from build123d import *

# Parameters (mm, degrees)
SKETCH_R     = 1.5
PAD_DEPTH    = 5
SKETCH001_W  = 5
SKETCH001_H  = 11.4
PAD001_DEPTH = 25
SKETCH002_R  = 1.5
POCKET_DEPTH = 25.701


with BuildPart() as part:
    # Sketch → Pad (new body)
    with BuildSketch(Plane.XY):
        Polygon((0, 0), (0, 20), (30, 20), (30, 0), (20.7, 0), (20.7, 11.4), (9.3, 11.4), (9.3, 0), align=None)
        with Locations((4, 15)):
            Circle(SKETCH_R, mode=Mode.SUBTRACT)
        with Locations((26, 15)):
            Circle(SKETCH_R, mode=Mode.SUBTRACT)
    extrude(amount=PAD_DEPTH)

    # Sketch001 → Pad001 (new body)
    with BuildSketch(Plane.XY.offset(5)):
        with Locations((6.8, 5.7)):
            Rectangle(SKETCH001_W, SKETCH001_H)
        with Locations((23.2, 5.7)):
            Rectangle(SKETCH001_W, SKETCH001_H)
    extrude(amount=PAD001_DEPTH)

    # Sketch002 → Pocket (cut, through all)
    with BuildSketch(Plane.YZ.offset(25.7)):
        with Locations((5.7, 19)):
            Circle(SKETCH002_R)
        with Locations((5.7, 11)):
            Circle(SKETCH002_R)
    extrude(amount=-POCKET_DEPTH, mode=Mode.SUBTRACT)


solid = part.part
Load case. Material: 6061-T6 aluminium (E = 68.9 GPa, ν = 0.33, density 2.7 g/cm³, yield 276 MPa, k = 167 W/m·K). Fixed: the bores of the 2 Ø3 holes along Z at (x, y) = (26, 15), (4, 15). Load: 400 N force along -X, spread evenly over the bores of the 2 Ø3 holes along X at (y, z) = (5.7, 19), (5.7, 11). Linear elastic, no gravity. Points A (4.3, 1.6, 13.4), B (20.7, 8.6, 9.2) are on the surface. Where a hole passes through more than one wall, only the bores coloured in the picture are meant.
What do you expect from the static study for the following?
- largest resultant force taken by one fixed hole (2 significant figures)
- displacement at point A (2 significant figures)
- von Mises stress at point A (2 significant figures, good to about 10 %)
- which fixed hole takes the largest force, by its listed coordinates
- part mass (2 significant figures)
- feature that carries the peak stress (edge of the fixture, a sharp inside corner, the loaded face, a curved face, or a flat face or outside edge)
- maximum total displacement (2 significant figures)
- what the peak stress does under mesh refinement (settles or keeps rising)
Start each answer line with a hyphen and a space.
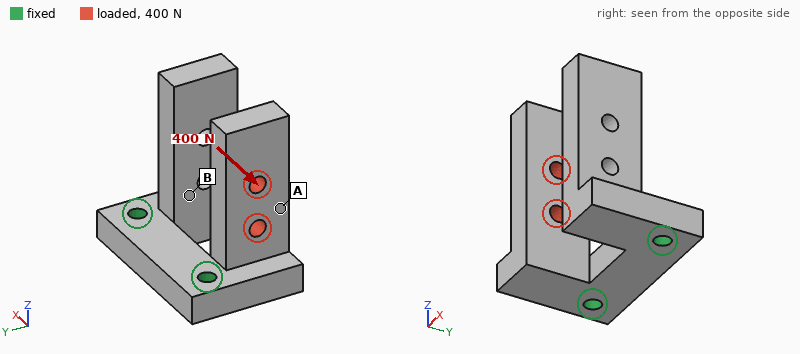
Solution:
- 380 N
- 0.074 mm
- 29 MPa
- (4, 15)
- 13 g
- a sharp inside corner
- 0.20 mm
- keeps rising
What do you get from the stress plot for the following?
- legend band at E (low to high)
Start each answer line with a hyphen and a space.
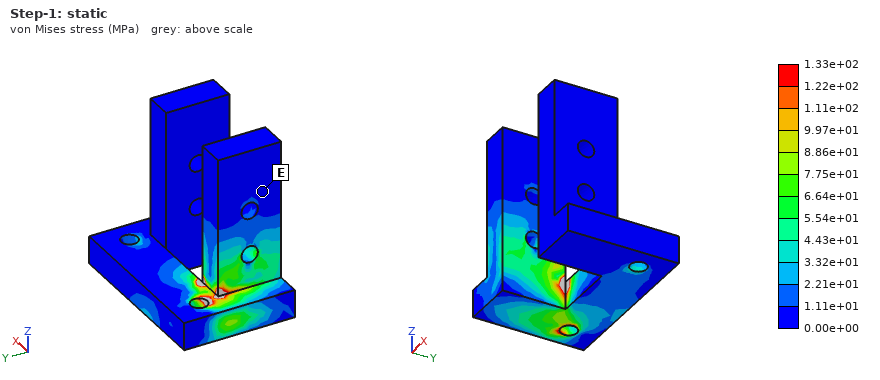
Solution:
- 0.00e+00 to 1.11e+01 MPa
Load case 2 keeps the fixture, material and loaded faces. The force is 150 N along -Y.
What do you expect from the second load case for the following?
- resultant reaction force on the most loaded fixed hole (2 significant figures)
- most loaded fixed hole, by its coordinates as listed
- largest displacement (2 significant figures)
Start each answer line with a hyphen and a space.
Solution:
- 140 N
- (4, 15)
- 59 µm
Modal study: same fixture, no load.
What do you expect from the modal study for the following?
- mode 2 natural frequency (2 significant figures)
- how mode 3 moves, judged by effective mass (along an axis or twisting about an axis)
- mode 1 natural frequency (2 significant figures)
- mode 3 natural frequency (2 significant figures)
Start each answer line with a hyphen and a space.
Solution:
- 3900 Hz
- along Y
- 3800 Hz
- 4400 Hz
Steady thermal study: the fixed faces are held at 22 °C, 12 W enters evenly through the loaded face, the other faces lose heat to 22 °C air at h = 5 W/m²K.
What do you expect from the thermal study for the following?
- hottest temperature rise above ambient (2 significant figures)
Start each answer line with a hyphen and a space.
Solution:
- 26 K
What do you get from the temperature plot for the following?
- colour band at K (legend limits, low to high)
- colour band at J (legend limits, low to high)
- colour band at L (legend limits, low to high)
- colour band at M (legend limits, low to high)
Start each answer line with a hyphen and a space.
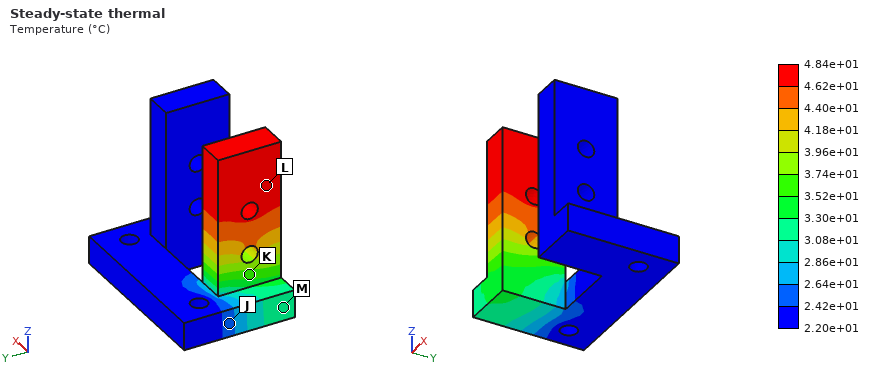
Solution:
- 3.52e+01 to 3.74e+01 °C
- 2.42e+01 to 2.64e+01 °C
- 4.62e+01 to 4.84e+01 °C
- 3.08e+01 to 3.30e+01 °C
